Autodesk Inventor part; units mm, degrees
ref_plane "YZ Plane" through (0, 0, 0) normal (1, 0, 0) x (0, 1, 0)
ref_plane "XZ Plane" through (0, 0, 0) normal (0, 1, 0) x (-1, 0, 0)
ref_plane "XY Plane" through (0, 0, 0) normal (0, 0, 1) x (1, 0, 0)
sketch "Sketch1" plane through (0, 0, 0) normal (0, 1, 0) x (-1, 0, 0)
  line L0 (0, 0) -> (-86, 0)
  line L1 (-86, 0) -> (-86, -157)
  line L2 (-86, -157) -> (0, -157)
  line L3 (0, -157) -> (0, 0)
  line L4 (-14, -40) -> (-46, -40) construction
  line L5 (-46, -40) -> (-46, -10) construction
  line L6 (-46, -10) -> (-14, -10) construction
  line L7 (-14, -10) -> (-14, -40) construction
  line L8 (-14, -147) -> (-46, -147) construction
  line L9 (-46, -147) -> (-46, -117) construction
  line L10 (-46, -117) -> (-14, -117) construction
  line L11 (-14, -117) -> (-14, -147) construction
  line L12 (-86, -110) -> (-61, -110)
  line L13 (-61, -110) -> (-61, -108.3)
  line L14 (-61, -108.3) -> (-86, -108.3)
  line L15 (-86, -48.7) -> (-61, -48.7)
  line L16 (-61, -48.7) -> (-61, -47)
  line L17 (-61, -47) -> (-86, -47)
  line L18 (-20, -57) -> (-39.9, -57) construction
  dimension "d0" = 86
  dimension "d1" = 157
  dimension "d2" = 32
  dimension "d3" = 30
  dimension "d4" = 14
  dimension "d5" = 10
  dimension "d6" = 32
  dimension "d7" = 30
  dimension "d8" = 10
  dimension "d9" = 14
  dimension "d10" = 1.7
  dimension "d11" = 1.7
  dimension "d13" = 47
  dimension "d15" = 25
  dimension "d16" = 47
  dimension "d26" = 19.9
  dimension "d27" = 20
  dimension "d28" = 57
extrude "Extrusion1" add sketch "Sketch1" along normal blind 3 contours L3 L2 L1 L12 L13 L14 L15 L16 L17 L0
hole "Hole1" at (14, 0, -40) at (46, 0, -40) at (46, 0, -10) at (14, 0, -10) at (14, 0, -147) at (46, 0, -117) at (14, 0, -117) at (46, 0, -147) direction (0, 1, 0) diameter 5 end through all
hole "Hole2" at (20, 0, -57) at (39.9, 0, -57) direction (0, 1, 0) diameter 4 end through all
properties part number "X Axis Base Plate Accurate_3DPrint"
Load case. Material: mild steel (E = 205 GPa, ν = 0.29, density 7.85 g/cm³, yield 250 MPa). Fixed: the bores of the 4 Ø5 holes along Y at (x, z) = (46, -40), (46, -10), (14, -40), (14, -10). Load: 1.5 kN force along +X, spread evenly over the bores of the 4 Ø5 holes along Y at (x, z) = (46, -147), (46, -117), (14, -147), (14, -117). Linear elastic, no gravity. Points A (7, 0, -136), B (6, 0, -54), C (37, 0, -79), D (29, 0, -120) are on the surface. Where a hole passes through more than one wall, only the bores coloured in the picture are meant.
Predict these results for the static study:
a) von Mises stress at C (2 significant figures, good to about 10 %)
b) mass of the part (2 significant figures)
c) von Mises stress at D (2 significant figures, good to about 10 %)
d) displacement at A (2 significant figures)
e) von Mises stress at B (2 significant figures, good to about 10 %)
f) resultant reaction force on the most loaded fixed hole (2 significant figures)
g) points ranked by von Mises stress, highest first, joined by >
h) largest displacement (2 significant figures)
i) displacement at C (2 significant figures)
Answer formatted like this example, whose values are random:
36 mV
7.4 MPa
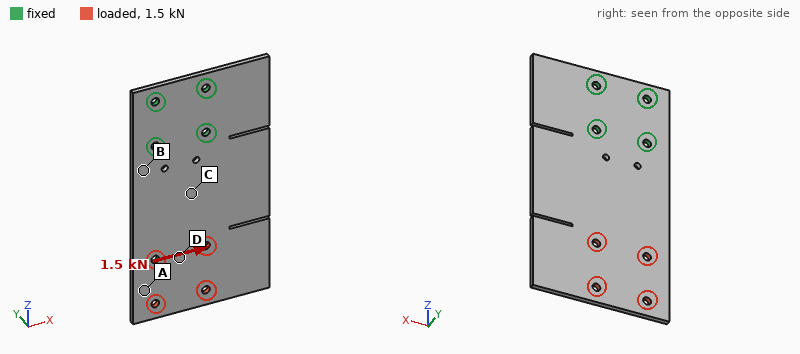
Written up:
22 MPa
310 g
14 MPa
52 µm
45 MPa
3.0 kN
B > C > D > A
69 µm
16 µm
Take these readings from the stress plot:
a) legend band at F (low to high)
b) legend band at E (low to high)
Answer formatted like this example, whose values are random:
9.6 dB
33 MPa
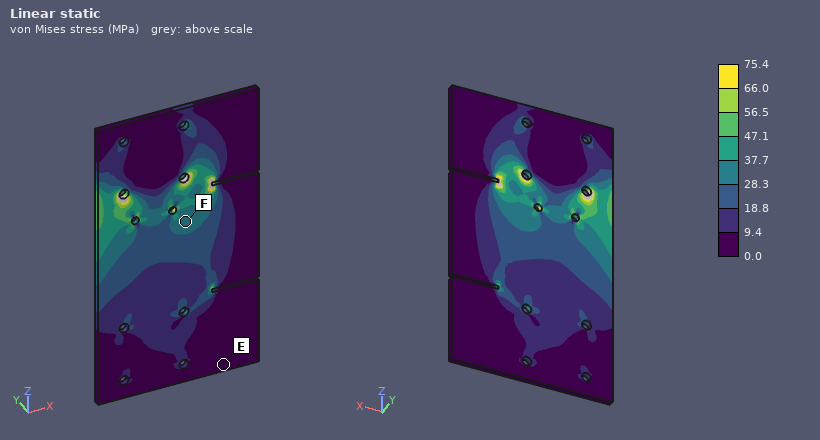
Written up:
28.3 to 37.7 MPa
0.0 to 9.4 MPa
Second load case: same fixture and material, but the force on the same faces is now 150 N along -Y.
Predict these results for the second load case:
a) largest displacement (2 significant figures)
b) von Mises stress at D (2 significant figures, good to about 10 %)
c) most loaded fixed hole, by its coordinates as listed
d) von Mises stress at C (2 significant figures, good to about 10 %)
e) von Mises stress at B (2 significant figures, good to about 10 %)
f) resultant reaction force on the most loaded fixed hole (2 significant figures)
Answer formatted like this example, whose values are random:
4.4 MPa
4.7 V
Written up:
1.7 mm
23 MPa
(46, -40)
62 MPa
120 MPa
160 N
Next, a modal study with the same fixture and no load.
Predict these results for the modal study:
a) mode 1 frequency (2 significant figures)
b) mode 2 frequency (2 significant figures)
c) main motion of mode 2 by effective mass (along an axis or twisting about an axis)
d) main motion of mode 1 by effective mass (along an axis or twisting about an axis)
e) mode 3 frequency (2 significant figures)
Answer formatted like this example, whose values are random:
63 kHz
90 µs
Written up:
160 Hz
480 Hz
twisting about Z
along Y
940 Hz
